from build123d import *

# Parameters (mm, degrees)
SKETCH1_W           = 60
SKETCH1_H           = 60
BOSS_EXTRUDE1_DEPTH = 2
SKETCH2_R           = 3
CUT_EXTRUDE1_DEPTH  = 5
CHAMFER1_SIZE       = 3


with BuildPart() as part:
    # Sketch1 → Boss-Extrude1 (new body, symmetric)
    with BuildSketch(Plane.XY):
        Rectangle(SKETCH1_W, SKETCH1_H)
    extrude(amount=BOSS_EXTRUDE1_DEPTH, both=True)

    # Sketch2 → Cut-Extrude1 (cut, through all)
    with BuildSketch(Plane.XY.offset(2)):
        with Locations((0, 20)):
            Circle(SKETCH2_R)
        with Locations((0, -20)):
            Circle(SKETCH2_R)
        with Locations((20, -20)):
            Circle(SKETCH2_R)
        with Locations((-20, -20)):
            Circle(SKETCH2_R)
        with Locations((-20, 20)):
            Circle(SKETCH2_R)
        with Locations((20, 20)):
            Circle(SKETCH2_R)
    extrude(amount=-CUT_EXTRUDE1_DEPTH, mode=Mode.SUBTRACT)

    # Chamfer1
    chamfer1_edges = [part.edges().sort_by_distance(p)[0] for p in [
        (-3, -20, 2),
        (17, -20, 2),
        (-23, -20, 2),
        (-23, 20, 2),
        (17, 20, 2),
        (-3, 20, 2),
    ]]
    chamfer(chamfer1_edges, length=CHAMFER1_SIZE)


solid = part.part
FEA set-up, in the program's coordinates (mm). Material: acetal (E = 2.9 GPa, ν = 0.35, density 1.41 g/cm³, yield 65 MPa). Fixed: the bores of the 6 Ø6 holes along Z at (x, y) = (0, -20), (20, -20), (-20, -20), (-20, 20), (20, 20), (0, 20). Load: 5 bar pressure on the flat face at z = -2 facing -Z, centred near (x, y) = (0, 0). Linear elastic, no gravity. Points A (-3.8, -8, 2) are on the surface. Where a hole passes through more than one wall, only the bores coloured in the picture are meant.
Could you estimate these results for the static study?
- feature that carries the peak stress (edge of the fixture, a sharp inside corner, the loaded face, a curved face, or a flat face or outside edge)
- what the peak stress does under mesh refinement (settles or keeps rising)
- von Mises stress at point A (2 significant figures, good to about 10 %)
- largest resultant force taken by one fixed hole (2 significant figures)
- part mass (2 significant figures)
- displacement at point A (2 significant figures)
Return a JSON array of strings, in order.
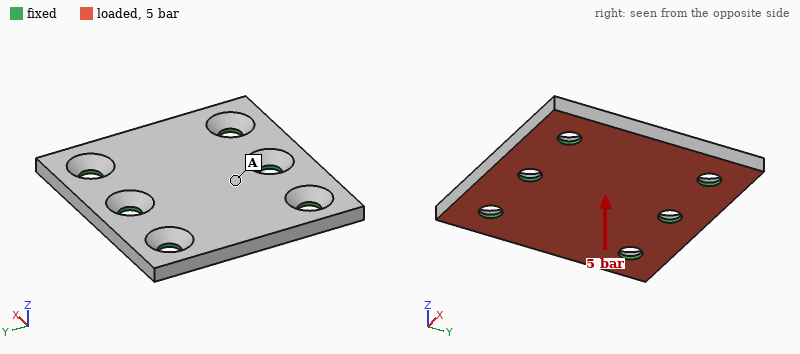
["edge of the fixture", "keeps rising", "10 MPa", "360 N", "18 g", "0.21 mm"]
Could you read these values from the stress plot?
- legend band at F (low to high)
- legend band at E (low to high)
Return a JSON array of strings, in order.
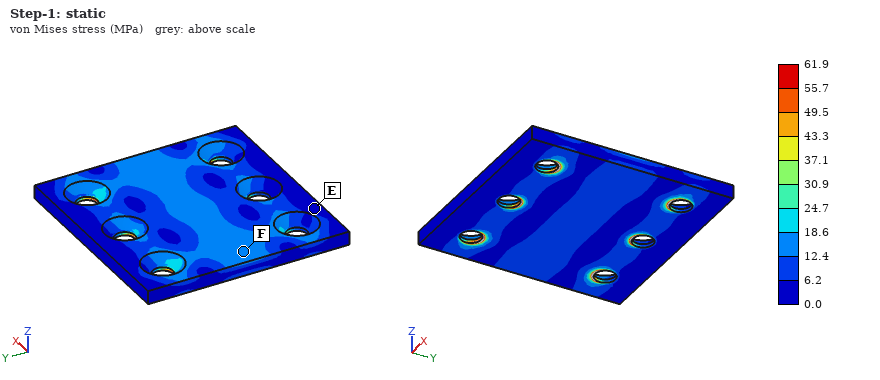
["12.4 to 18.6 MPa", "0.0 to 6.2 MPa"]
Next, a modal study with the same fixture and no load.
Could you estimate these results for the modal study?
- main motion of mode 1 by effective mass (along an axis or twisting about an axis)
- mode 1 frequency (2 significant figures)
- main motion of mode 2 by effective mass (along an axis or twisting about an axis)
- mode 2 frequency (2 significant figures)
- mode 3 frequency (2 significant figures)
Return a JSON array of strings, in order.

["along Z", "2800 Hz", "twisting about Y", "3000 Hz", "4000 Hz"]
